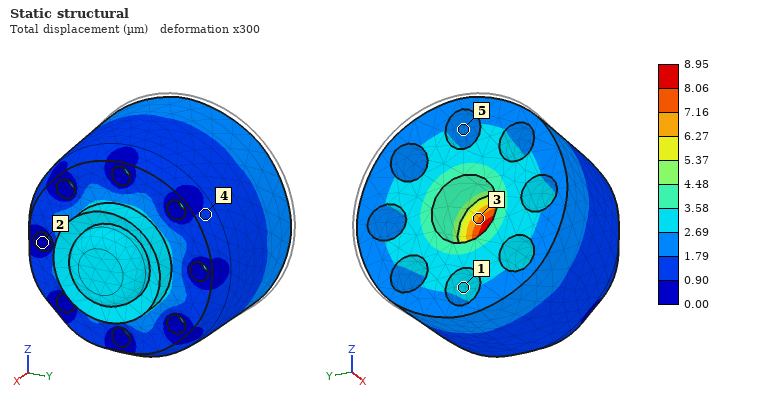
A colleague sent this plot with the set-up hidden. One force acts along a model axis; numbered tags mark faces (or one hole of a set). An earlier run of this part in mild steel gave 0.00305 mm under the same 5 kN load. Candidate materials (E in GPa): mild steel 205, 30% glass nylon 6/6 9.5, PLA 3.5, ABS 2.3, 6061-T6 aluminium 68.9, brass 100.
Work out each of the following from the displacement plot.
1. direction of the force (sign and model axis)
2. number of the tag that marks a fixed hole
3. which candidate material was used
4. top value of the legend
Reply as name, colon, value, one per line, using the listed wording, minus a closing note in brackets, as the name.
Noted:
direction of the force: +X
number of the tag that marks a fixed hole: 2
which candidate material was used: 6061-T6 aluminium
top value of the legend: 8.95 µm
